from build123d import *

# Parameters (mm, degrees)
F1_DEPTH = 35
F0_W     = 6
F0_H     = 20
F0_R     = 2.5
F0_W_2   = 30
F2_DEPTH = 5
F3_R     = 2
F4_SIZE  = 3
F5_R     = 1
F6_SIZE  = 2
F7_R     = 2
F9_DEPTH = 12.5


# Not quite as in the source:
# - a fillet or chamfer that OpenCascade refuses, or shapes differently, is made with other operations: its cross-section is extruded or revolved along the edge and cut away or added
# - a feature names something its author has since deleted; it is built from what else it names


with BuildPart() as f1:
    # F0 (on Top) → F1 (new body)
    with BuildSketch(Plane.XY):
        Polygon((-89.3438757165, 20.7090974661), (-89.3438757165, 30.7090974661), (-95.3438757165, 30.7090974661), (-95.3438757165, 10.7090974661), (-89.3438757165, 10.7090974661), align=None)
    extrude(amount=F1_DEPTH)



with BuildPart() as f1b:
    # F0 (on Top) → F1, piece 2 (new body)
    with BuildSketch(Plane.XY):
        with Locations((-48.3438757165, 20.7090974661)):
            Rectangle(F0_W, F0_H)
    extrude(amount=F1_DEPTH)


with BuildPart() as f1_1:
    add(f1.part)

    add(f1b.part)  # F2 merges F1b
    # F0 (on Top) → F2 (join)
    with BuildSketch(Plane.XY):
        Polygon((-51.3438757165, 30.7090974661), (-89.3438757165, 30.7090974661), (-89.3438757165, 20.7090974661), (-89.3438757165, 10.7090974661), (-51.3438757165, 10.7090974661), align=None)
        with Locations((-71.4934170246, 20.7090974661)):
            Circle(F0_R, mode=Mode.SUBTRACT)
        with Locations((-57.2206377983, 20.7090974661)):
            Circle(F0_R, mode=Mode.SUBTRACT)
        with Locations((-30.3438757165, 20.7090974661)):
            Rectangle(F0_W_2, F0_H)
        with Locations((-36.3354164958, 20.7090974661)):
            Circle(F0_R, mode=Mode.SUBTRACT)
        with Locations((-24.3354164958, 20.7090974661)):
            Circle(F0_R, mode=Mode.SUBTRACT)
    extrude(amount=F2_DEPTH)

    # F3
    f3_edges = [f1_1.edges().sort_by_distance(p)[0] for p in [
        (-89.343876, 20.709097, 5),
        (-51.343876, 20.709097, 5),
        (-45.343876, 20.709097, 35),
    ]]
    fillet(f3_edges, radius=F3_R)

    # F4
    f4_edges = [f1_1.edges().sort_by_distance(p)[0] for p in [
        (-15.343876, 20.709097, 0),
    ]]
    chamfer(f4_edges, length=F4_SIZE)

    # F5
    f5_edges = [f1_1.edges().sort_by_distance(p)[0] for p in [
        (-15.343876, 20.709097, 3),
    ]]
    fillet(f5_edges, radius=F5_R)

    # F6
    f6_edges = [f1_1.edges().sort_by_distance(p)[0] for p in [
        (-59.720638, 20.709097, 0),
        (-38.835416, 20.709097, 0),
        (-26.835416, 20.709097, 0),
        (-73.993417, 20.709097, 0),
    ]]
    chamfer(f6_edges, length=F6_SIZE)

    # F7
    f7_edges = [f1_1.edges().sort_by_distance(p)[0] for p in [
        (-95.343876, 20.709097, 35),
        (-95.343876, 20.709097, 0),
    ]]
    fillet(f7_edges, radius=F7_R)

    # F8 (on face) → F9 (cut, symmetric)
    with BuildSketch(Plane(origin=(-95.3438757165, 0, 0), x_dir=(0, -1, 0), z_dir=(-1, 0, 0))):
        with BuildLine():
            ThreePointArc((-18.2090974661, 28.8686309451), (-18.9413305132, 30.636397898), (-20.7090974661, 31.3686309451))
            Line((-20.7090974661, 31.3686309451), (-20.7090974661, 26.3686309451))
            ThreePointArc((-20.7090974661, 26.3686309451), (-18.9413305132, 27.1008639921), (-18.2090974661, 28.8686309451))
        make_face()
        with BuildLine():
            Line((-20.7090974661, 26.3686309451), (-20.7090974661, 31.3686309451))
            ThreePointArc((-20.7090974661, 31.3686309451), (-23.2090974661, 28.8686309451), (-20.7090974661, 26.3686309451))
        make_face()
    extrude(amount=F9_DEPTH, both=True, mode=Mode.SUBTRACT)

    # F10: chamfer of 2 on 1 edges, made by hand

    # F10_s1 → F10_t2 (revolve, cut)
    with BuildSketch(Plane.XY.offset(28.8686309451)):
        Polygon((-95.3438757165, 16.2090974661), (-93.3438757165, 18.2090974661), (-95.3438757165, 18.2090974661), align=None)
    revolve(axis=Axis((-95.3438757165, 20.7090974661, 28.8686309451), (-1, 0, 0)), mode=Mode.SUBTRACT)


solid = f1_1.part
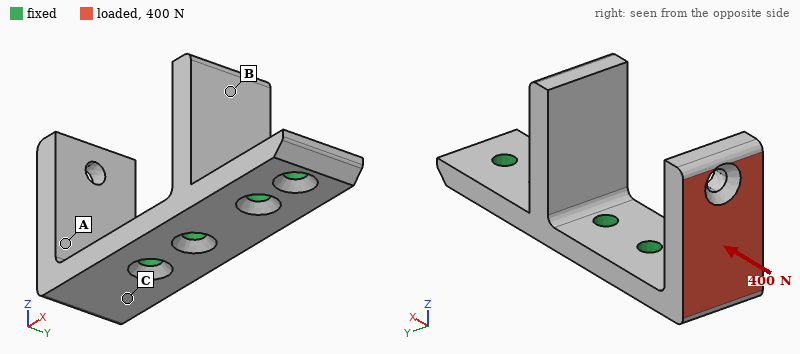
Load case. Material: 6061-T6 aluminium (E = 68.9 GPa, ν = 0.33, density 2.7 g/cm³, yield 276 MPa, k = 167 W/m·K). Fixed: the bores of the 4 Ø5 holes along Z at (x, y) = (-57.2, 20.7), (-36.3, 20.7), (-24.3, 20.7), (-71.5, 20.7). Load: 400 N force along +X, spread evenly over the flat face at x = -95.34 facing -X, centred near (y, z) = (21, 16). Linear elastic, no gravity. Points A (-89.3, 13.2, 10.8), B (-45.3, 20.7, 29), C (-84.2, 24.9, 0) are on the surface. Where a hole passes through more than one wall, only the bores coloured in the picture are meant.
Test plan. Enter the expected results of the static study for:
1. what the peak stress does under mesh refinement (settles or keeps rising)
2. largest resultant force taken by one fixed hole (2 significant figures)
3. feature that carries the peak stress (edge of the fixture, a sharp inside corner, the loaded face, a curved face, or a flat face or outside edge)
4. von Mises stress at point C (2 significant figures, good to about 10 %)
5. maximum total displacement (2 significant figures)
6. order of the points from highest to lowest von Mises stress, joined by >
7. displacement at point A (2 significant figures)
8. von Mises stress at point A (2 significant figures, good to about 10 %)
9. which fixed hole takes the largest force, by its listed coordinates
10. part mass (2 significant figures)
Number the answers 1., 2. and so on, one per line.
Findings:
1. keeps rising
2. 530 N
3. edge of the fixture
4. 57 MPa
5. 0.31 mm
6. C > A > B
7. 0.093 mm
8. 21 MPa
9. (-71.5, 20.7)
10. 39 g
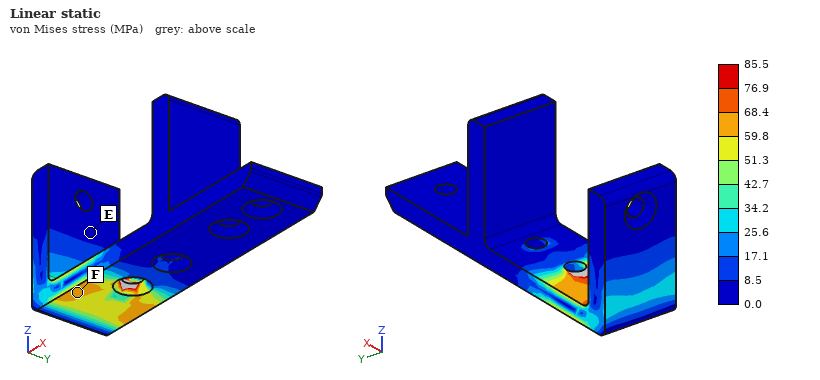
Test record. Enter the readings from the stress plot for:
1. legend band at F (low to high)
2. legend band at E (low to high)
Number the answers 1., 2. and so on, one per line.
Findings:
1. 59.8 to 68.4 MPa
2. 0.0 to 8.5 MPa
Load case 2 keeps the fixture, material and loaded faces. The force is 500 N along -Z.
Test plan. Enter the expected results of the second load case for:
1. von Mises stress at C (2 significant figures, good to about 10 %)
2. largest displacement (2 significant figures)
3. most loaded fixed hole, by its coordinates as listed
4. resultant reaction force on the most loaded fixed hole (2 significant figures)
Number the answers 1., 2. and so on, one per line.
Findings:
1. 61 MPa
2. 0.39 mm
3. (-71.5, 20.7)
4. 920 N
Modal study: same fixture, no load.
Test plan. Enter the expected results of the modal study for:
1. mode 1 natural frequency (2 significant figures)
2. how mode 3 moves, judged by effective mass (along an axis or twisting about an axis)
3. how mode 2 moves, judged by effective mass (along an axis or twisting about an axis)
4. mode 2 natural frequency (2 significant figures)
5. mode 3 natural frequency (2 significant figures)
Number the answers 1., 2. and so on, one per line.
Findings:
1. 1800 Hz
2. along X
3. along Y
4. 2500 Hz
5. 4600 Hz
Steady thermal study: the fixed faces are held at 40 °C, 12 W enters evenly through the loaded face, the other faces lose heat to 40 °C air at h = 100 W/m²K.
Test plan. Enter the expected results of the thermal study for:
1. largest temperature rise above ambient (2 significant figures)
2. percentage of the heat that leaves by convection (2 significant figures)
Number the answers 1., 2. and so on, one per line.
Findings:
1. 18 K
2. 23 %
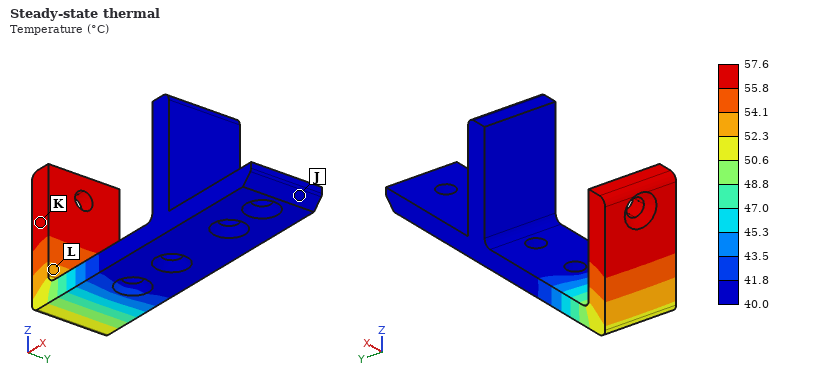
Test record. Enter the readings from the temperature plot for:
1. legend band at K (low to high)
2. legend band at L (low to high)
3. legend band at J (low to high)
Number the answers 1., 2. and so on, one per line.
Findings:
1. 55.8 to 57.6 °C
2. 52.3 to 54.1 °C
3. 40.0 to 41.8 °C
